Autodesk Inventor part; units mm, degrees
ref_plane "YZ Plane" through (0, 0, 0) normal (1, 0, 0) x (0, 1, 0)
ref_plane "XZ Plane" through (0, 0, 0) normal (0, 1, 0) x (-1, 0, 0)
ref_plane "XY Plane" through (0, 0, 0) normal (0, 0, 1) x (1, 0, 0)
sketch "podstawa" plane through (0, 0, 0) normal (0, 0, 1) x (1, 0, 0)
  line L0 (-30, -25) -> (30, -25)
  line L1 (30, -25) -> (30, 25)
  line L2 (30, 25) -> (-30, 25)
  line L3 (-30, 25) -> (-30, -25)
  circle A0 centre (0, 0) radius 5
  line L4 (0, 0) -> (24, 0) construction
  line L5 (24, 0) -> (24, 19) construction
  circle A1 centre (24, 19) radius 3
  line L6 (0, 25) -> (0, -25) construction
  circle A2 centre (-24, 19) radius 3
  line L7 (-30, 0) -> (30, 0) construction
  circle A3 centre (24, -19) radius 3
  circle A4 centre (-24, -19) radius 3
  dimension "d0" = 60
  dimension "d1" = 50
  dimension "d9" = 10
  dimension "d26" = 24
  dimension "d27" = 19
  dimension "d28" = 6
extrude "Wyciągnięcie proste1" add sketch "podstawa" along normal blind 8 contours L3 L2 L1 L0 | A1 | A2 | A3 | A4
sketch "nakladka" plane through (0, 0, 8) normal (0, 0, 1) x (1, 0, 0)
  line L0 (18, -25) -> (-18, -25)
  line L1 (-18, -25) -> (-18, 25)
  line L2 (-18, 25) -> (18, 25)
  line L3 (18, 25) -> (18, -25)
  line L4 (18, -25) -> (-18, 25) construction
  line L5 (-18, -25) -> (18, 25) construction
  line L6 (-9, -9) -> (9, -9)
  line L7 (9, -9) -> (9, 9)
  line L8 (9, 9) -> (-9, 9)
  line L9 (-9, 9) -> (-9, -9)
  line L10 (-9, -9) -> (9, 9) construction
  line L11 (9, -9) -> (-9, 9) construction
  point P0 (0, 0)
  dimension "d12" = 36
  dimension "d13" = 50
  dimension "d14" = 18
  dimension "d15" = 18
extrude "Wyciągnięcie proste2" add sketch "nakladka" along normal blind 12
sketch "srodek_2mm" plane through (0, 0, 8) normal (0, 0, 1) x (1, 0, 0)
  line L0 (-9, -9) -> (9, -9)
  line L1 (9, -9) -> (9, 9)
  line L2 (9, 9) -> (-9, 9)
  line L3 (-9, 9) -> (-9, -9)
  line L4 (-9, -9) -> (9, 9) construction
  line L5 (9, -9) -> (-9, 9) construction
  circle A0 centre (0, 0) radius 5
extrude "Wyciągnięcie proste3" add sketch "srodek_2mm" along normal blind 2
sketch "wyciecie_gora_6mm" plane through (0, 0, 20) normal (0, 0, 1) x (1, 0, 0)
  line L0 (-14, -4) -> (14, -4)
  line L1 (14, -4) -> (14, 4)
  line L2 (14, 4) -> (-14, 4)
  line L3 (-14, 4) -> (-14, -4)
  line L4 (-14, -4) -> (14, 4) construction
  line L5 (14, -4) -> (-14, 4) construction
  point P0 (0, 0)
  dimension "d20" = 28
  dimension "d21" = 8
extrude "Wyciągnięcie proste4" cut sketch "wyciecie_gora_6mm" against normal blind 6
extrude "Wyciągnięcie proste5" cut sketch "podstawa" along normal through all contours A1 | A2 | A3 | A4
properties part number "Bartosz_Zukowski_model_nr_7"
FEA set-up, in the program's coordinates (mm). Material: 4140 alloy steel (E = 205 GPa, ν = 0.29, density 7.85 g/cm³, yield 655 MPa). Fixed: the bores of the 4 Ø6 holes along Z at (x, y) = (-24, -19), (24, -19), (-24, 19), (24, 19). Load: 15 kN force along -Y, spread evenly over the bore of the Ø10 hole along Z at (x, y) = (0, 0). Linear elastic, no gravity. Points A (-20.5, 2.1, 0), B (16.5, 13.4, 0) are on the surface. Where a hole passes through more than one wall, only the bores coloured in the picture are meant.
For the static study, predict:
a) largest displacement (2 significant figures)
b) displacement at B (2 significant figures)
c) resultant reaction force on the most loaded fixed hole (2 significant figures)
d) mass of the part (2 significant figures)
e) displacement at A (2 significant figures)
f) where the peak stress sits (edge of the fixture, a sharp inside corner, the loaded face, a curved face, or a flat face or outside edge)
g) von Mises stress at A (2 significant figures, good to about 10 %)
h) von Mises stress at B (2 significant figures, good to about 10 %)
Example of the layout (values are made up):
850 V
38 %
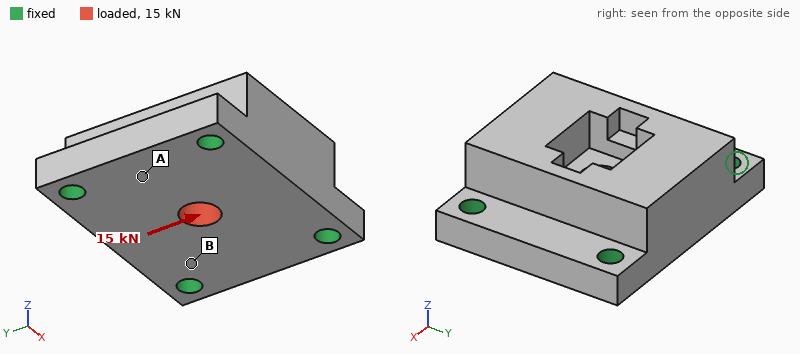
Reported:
6.1 µm
1.9 µm
4.2 kN
320 g
1.6 µm
edge of the fixture
19 MPa
38 MPa
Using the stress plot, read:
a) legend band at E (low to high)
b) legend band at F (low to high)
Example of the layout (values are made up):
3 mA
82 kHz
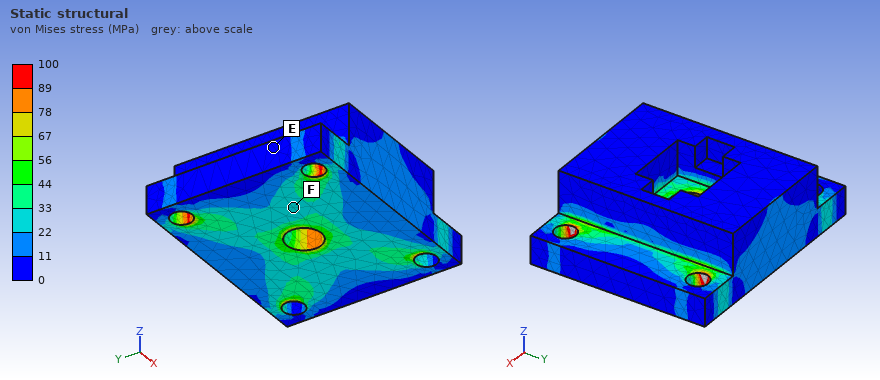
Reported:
0 to 11 MPa
22 to 33 MPa
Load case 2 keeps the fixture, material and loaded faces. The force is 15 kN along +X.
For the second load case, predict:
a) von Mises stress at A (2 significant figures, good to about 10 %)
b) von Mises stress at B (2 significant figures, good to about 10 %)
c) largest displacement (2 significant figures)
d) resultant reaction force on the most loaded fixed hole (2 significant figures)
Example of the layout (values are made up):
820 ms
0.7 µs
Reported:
10 MPa
34 MPa
4.8 µm
4.0 kN
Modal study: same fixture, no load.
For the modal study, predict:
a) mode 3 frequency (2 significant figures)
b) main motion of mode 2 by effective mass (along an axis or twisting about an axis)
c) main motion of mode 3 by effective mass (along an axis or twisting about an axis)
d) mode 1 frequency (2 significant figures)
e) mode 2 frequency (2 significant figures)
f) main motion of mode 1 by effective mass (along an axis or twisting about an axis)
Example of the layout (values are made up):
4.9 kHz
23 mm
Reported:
23 kHz
along Y
along Y
16 kHz
17 kHz
along Z
